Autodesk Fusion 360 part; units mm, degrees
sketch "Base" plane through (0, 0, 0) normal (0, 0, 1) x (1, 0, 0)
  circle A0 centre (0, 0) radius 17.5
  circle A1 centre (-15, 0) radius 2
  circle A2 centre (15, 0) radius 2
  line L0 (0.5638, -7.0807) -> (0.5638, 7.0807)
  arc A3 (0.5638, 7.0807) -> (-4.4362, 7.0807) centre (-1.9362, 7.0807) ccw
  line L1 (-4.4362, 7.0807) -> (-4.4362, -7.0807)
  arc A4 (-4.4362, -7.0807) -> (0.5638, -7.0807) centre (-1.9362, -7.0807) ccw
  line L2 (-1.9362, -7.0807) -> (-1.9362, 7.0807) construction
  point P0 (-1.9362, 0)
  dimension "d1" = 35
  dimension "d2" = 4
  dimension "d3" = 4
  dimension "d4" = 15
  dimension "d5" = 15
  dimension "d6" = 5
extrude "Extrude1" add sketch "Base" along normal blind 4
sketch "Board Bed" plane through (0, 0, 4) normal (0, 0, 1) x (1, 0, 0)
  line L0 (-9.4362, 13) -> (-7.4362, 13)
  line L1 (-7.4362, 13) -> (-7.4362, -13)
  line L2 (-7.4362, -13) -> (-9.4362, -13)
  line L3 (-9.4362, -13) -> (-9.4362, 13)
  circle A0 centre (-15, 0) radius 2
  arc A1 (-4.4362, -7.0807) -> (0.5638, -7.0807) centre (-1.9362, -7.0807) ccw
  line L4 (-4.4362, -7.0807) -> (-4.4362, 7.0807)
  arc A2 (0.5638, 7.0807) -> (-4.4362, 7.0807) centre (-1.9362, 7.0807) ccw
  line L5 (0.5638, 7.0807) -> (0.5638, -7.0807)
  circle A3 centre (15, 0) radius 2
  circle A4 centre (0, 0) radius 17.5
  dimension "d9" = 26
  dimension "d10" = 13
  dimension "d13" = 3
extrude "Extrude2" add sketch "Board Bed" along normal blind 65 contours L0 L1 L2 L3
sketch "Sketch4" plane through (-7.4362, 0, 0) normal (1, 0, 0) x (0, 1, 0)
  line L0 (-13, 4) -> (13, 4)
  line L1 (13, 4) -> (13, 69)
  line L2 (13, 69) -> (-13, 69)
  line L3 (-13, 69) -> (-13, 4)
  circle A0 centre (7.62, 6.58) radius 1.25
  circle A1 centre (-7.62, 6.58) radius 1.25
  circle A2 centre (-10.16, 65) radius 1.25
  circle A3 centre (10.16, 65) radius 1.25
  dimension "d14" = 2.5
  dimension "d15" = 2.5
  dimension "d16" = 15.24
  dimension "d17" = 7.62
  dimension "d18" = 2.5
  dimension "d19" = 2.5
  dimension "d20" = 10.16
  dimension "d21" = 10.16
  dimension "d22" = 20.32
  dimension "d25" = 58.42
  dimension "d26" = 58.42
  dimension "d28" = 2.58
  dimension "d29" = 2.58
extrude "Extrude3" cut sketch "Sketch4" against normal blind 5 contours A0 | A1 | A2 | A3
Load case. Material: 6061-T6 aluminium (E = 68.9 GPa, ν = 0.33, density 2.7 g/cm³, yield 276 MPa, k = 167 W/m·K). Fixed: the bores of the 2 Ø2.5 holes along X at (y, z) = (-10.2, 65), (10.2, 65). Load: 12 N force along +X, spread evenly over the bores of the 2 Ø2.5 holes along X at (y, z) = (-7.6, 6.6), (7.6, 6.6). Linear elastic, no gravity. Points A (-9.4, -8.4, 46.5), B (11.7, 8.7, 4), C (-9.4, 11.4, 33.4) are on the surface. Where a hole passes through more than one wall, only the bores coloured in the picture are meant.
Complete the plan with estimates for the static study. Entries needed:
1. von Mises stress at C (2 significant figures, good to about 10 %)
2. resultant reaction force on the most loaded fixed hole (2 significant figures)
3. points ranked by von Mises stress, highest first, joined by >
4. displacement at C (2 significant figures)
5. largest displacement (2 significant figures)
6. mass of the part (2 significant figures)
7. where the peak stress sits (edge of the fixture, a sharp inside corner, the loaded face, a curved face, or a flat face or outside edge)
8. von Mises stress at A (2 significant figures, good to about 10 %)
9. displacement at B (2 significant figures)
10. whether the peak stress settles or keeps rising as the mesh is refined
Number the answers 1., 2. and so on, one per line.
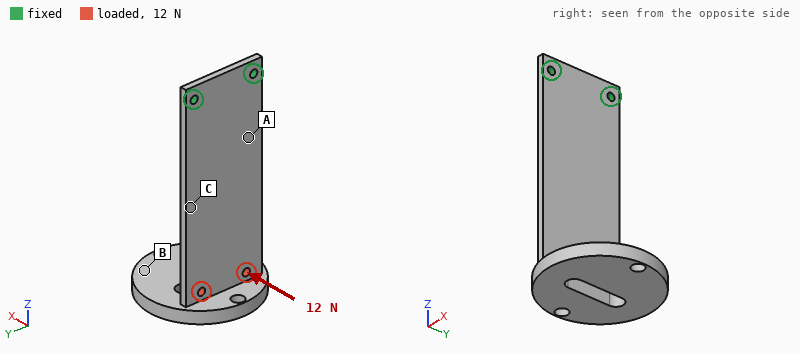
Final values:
1. 19 MPa
2. 6.0 N
3. A > C > B
4. 0.25 mm
5. 0.92 mm
6. 18 g
7. edge of the fixture
8. 27 MPa
9. 0.81 mm
10. keeps rising
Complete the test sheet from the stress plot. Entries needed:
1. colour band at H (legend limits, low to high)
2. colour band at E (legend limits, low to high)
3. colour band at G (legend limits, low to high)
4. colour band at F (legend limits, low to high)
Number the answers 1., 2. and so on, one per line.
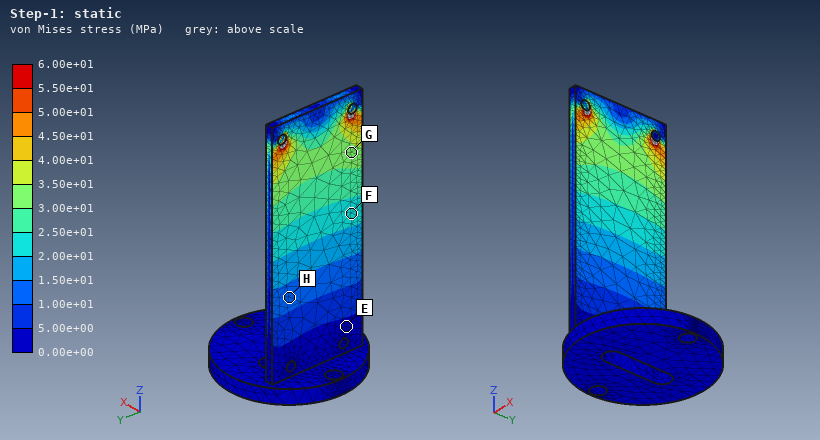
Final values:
1. 1.00e+01 to 1.50e+01 MPa
2. 0.00e+00 to 5.00e+00 MPa
3. 3.00e+01 to 3.50e+01 MPa
4. 2.00e+01 to 2.50e+01 MPa
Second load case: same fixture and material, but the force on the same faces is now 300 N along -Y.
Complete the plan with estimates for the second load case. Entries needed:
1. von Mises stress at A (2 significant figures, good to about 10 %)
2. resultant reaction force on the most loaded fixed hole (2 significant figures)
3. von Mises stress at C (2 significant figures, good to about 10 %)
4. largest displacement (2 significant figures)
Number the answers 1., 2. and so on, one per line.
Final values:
1. 36 MPa
2. 850 N
3. 32 MPa
4. 0.14 mm
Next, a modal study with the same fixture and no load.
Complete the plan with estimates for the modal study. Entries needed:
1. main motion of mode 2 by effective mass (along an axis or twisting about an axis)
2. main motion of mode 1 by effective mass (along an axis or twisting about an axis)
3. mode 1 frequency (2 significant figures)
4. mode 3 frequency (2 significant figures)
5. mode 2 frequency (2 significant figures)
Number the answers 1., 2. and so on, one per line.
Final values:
1. along Y
2. along X
3. 170 Hz
4. 1000 Hz
5. 610 Hz
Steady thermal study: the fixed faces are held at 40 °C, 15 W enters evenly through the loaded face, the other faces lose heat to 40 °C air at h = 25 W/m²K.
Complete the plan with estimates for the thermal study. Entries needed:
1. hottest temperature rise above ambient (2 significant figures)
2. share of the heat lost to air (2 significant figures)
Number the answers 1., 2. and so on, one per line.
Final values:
1. 68 K
2. 43 %
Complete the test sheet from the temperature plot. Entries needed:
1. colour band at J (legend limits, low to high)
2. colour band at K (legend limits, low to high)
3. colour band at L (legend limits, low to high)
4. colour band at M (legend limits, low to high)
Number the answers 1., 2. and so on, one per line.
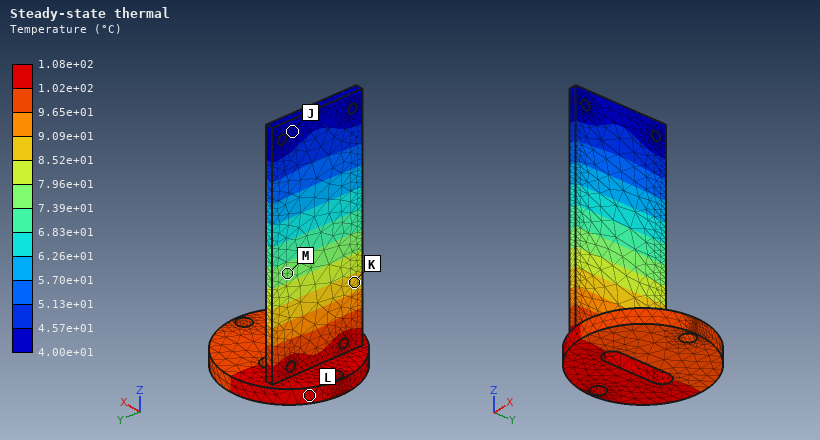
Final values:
1. 4.00e+01 to 4.57e+01 °C
2. 8.52e+01 to 9.09e+01 °C
3. 1.02e+02 to 1.08e+02 °C
4. 7.39e+01 to 7.96e+01 °C
